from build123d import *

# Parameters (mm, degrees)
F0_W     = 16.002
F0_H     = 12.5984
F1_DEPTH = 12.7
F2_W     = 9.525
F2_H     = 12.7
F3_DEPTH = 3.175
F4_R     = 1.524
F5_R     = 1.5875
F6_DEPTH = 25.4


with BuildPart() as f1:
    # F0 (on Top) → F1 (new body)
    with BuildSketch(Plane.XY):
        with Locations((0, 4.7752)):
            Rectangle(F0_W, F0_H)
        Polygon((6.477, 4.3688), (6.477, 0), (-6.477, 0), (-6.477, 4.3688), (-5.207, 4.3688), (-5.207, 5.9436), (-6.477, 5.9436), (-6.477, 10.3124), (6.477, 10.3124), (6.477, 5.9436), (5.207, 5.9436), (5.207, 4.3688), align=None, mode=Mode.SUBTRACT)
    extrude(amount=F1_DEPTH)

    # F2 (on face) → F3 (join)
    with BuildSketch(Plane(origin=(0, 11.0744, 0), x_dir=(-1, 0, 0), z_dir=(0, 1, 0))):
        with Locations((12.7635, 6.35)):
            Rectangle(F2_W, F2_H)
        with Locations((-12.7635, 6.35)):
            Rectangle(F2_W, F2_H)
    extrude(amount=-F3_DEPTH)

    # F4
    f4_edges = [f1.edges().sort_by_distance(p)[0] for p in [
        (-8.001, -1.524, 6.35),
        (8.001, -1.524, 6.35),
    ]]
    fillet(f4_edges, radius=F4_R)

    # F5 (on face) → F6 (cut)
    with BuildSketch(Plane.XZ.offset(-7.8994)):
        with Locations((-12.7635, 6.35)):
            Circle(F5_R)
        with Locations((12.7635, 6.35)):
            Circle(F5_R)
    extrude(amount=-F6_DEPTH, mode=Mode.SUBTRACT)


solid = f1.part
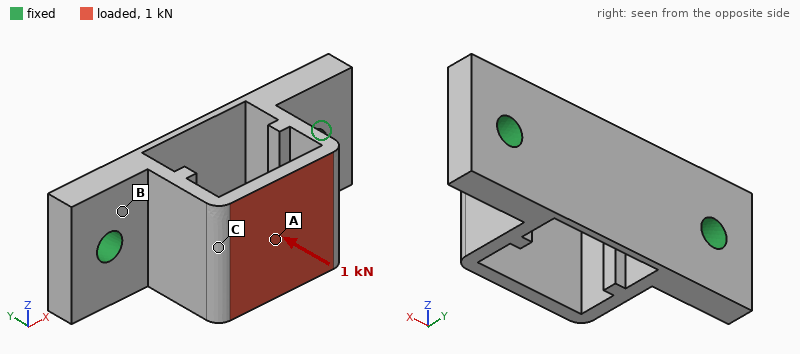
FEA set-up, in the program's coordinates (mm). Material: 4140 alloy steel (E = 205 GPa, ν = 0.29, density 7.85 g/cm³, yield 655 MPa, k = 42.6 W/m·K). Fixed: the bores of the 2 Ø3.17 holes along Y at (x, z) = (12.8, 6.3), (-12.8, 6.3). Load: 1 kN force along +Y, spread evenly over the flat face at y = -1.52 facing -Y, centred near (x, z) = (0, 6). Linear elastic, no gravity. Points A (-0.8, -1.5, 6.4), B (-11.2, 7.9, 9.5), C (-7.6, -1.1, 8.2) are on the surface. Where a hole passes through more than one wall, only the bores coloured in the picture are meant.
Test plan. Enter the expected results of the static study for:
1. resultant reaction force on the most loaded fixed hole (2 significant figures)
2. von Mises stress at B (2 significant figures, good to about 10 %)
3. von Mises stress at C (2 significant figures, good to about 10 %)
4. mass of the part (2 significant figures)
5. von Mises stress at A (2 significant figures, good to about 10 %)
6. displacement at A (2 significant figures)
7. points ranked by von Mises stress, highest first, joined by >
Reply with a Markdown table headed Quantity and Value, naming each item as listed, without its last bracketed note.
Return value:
| Quantity | Value |
|---|---|
| resultant reaction force on the most loaded fixed hole | 500 N |
| von Mises stress at B | 25 MPa |
| von Mises stress at C | 72 MPa |
| mass of the part | 13 g |
| von Mises stress at A | 170 MPa |
| displacement at A | 23 µm |
| points ranked by von Mises stress, highest first, joined by > | A > C > B |
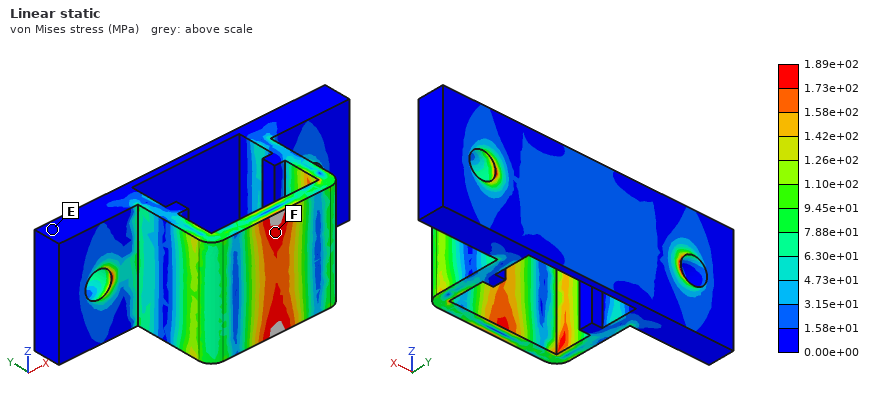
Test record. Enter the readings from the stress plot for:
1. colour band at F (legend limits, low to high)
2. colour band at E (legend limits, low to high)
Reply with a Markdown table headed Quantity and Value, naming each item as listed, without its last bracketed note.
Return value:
| Quantity | Value |
|---|---|
| colour band at F | 1.73e+02 to 1.89e+02 MPa |
| colour band at E | 0.00e+00 to 1.58e+01 MPa |
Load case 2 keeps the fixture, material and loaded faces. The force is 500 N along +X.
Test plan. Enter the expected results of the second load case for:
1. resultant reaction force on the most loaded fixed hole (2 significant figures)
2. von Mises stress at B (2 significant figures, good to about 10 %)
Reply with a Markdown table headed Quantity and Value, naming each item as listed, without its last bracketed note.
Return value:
| Quantity | Value |
|---|---|
| resultant reaction force on the most loaded fixed hole | 300 N |
| von Mises stress at B | 35 MPa |
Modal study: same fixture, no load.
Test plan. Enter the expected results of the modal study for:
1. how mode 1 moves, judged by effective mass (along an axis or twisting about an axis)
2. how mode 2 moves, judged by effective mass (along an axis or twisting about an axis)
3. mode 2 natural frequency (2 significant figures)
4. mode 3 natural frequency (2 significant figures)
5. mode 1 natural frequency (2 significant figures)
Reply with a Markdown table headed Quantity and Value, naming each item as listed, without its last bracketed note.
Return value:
| Quantity | Value |
|---|---|
| how mode 1 moves, judged by effective mass | along X |
| how mode 2 moves, judged by effective mass | along Z |
| mode 2 natural frequency | 14 kHz |
| mode 3 natural frequency | 18 kHz |
| mode 1 natural frequency | 10 kHz |
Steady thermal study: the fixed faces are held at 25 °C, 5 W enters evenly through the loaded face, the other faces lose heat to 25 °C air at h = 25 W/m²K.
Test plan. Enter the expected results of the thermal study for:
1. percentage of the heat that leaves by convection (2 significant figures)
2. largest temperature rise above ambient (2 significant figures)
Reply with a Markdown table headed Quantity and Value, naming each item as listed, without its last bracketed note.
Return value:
| Quantity | Value |
|---|---|
| percentage of the heat that leaves by convection | 12 % |
| largest temperature rise above ambient | 43 K |
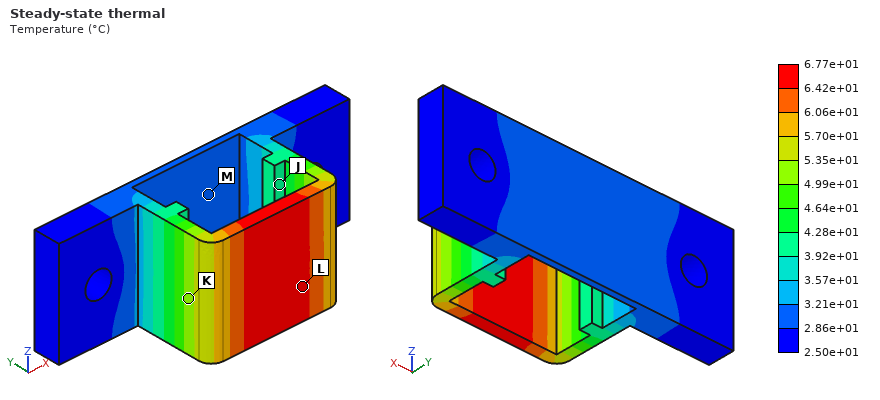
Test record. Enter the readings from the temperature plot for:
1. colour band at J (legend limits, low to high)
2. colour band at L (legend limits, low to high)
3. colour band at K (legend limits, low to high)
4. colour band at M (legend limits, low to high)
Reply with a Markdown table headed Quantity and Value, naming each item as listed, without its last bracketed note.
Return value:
| Quantity | Value |
|---|---|
| colour band at J | 3.92e+01 to 4.28e+01 °C |
| colour band at L | 6.42e+01 to 6.77e+01 °C |
| colour band at K | 4.99e+01 to 5.35e+01 °C |
| colour band at M | 2.86e+01 to 3.21e+01 °C |
